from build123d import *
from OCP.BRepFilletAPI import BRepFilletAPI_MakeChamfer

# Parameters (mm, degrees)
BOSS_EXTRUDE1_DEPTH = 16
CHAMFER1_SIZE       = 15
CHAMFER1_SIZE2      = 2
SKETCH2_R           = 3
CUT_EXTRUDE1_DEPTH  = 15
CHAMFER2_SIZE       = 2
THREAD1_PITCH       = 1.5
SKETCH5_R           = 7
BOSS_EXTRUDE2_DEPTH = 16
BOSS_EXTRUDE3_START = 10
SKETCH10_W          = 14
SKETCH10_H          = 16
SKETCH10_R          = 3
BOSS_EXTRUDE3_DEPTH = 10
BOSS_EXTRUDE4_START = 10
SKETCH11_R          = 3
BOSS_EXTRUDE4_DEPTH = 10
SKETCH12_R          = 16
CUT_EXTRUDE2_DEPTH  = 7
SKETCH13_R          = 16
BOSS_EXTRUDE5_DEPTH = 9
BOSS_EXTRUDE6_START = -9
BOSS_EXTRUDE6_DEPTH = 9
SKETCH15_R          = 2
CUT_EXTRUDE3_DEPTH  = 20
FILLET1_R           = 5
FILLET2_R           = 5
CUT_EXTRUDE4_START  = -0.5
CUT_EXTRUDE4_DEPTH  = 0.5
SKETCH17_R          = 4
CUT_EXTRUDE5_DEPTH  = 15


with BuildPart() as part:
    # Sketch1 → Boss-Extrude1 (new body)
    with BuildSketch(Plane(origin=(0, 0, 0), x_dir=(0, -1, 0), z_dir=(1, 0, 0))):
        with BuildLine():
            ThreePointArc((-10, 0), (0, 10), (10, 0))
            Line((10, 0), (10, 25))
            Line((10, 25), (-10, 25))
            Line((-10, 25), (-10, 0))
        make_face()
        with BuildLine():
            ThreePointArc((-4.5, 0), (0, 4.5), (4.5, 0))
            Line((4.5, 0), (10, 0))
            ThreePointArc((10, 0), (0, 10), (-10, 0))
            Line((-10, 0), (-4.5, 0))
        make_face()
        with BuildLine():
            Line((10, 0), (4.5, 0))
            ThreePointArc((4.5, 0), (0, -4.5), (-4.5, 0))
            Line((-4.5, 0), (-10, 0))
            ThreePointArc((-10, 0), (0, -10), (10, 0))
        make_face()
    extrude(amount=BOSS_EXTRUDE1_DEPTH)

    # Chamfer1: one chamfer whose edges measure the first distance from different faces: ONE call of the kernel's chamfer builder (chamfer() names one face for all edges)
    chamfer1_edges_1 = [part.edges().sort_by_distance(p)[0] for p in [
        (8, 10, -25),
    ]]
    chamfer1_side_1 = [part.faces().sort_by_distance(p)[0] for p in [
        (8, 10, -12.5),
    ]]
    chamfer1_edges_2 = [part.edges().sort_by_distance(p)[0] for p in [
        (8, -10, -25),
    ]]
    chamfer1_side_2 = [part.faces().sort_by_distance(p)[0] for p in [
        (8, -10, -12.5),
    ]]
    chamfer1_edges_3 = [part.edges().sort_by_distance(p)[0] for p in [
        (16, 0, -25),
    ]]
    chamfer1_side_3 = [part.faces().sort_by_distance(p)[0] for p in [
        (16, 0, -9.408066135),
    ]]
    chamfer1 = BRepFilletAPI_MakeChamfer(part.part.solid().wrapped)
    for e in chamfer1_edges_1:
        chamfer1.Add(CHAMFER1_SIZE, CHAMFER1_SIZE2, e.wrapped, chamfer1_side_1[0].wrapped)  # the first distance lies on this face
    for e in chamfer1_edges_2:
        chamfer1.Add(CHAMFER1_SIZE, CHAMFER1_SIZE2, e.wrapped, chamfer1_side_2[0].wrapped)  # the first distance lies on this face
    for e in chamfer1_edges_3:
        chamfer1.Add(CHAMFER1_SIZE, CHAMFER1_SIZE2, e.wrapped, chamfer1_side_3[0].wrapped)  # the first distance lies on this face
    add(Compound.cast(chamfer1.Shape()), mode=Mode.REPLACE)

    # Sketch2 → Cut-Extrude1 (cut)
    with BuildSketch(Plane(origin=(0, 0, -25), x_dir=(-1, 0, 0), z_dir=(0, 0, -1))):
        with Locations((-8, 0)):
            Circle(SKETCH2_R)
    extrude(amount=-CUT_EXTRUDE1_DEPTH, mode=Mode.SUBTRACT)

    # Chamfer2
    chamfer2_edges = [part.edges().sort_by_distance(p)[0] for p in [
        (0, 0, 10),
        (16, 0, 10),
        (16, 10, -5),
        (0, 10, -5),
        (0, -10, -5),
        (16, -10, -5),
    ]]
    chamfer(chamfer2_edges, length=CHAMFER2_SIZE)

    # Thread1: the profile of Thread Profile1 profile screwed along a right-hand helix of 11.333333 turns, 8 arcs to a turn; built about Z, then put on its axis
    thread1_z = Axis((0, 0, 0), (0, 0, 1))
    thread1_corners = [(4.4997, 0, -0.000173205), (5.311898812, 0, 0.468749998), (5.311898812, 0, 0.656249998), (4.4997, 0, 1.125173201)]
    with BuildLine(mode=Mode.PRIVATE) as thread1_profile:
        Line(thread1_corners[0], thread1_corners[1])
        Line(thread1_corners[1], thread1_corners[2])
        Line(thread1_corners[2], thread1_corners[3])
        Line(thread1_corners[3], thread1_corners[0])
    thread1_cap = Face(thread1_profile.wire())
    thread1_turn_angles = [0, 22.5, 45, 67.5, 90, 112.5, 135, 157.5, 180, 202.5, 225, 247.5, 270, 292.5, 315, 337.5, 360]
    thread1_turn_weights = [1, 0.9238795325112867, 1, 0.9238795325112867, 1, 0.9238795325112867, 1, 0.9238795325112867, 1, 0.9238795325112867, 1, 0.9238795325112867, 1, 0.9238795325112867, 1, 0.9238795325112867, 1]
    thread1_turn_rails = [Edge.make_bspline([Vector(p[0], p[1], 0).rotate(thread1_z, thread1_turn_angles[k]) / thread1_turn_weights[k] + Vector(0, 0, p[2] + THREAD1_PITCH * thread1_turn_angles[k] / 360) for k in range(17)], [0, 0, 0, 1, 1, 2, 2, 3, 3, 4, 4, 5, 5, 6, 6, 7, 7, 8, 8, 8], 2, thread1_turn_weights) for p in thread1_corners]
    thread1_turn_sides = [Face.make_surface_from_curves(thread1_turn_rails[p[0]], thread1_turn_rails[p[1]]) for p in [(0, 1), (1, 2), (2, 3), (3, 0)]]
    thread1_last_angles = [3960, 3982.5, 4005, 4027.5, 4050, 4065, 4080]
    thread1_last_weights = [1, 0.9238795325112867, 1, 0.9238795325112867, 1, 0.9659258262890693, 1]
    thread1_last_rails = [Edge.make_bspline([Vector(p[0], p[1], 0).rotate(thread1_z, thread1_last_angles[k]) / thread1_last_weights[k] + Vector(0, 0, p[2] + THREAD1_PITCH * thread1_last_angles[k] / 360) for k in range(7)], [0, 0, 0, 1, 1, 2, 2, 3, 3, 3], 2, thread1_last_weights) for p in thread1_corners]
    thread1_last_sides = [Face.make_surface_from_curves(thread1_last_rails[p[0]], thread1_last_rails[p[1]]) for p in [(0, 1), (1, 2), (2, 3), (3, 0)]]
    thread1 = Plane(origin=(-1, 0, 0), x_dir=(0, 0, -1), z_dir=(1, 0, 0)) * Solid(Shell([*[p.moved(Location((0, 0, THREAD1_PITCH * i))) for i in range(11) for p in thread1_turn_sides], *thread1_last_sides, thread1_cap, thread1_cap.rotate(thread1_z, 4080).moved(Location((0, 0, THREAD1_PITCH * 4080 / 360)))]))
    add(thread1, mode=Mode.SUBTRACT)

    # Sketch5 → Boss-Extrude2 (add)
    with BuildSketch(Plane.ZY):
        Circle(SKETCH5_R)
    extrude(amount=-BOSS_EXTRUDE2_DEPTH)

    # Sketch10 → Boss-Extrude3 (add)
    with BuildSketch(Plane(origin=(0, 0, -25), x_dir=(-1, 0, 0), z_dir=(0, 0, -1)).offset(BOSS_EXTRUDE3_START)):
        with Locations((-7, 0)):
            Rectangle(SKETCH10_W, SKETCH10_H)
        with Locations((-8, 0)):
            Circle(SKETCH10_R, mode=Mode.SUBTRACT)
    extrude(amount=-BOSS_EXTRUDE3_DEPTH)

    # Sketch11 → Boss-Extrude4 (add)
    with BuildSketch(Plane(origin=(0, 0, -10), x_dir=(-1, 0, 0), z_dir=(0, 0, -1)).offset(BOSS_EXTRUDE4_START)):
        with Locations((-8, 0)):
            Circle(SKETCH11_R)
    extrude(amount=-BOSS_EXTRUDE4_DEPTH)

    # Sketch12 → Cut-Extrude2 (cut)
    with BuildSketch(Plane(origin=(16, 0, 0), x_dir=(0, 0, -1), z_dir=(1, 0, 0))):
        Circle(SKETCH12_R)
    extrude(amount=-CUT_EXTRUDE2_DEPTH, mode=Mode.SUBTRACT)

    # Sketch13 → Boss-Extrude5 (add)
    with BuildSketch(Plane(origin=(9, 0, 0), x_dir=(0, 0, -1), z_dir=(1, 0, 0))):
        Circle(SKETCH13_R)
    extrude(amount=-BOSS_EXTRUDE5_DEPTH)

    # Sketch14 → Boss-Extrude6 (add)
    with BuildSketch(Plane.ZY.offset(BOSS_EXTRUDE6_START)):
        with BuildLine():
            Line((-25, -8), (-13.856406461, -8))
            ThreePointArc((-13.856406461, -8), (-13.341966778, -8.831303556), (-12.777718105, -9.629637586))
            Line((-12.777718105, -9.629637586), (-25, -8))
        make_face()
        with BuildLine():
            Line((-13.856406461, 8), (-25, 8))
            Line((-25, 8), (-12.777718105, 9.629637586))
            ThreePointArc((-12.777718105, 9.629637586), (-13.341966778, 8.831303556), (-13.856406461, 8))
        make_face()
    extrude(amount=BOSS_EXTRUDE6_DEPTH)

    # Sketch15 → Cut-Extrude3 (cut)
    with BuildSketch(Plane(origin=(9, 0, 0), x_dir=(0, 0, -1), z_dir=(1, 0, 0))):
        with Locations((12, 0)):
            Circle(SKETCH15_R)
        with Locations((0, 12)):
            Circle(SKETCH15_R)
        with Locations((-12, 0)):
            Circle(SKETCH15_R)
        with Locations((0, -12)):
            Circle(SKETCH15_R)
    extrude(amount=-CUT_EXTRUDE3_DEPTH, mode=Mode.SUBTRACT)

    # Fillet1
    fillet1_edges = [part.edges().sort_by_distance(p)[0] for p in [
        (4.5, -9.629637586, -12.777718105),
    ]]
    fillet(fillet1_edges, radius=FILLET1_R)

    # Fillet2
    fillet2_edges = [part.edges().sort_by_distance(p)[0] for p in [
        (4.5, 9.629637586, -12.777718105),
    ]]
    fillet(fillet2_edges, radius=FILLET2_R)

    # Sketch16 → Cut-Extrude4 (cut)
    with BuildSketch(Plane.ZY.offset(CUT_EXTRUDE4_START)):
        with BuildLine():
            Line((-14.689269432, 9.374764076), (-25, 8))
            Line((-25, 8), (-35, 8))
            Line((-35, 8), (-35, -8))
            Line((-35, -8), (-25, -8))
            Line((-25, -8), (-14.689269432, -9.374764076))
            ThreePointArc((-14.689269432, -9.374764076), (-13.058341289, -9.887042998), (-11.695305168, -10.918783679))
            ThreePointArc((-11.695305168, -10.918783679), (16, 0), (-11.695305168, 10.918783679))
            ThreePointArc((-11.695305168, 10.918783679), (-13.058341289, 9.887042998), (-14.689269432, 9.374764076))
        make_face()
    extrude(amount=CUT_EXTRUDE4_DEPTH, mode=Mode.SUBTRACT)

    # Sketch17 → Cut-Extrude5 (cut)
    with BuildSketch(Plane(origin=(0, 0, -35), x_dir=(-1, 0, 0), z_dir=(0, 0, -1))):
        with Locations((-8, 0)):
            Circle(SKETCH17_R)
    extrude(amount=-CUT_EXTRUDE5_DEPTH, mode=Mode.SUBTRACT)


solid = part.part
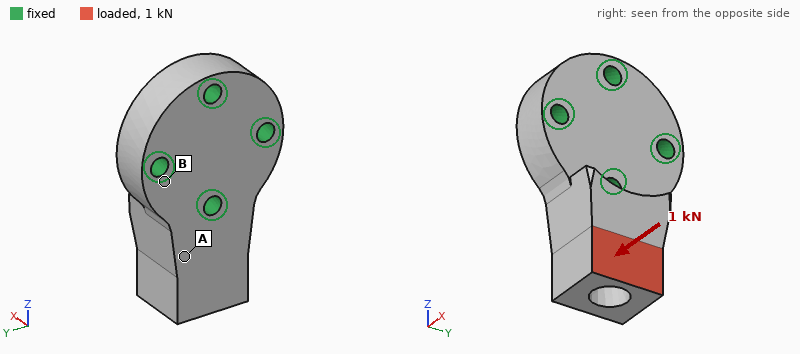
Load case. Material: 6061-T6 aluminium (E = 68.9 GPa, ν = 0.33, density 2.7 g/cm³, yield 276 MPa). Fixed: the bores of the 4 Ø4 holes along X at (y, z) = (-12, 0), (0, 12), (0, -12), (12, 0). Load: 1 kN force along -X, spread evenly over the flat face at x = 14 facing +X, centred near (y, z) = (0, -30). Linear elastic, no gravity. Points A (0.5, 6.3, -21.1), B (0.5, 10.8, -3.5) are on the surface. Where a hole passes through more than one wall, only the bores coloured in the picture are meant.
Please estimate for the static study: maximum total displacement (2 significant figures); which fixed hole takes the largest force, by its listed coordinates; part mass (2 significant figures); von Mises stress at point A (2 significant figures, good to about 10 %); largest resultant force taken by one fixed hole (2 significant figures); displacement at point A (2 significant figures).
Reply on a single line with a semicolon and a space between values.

48 µm; (0, -12); 28 g; 26 MPa; 1.4 kN; 15 µm
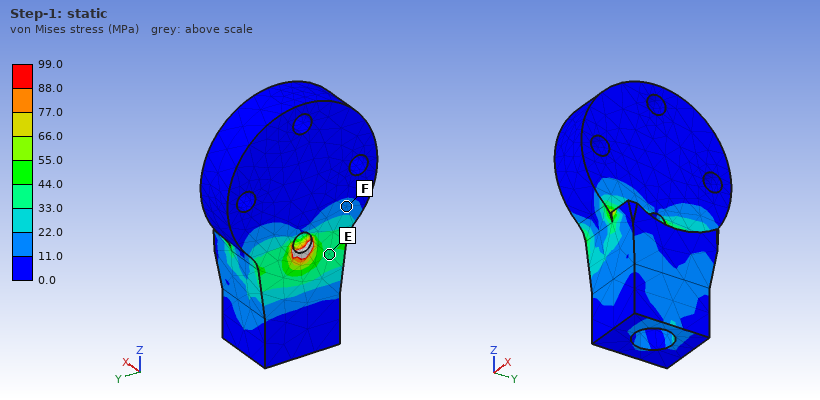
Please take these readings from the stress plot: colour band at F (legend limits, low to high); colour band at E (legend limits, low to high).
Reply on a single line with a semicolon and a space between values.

11.0 to 22.0 MPa; 33.0 to 44.0 MPa
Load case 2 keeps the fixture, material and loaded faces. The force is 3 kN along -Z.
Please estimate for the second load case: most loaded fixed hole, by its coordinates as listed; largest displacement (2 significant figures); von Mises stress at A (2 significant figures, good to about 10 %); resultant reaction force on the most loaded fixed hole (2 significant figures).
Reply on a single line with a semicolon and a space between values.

(0, -12); 87 µm; 42 MPa; 2.1 kN
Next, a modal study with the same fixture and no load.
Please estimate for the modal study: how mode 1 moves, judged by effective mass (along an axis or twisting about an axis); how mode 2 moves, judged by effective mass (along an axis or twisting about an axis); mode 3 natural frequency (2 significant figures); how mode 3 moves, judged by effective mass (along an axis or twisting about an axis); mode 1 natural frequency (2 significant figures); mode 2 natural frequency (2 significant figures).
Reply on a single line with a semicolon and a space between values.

along X; along Y; 23 kHz; twisting about Z; 11 kHz; 17 kHz
